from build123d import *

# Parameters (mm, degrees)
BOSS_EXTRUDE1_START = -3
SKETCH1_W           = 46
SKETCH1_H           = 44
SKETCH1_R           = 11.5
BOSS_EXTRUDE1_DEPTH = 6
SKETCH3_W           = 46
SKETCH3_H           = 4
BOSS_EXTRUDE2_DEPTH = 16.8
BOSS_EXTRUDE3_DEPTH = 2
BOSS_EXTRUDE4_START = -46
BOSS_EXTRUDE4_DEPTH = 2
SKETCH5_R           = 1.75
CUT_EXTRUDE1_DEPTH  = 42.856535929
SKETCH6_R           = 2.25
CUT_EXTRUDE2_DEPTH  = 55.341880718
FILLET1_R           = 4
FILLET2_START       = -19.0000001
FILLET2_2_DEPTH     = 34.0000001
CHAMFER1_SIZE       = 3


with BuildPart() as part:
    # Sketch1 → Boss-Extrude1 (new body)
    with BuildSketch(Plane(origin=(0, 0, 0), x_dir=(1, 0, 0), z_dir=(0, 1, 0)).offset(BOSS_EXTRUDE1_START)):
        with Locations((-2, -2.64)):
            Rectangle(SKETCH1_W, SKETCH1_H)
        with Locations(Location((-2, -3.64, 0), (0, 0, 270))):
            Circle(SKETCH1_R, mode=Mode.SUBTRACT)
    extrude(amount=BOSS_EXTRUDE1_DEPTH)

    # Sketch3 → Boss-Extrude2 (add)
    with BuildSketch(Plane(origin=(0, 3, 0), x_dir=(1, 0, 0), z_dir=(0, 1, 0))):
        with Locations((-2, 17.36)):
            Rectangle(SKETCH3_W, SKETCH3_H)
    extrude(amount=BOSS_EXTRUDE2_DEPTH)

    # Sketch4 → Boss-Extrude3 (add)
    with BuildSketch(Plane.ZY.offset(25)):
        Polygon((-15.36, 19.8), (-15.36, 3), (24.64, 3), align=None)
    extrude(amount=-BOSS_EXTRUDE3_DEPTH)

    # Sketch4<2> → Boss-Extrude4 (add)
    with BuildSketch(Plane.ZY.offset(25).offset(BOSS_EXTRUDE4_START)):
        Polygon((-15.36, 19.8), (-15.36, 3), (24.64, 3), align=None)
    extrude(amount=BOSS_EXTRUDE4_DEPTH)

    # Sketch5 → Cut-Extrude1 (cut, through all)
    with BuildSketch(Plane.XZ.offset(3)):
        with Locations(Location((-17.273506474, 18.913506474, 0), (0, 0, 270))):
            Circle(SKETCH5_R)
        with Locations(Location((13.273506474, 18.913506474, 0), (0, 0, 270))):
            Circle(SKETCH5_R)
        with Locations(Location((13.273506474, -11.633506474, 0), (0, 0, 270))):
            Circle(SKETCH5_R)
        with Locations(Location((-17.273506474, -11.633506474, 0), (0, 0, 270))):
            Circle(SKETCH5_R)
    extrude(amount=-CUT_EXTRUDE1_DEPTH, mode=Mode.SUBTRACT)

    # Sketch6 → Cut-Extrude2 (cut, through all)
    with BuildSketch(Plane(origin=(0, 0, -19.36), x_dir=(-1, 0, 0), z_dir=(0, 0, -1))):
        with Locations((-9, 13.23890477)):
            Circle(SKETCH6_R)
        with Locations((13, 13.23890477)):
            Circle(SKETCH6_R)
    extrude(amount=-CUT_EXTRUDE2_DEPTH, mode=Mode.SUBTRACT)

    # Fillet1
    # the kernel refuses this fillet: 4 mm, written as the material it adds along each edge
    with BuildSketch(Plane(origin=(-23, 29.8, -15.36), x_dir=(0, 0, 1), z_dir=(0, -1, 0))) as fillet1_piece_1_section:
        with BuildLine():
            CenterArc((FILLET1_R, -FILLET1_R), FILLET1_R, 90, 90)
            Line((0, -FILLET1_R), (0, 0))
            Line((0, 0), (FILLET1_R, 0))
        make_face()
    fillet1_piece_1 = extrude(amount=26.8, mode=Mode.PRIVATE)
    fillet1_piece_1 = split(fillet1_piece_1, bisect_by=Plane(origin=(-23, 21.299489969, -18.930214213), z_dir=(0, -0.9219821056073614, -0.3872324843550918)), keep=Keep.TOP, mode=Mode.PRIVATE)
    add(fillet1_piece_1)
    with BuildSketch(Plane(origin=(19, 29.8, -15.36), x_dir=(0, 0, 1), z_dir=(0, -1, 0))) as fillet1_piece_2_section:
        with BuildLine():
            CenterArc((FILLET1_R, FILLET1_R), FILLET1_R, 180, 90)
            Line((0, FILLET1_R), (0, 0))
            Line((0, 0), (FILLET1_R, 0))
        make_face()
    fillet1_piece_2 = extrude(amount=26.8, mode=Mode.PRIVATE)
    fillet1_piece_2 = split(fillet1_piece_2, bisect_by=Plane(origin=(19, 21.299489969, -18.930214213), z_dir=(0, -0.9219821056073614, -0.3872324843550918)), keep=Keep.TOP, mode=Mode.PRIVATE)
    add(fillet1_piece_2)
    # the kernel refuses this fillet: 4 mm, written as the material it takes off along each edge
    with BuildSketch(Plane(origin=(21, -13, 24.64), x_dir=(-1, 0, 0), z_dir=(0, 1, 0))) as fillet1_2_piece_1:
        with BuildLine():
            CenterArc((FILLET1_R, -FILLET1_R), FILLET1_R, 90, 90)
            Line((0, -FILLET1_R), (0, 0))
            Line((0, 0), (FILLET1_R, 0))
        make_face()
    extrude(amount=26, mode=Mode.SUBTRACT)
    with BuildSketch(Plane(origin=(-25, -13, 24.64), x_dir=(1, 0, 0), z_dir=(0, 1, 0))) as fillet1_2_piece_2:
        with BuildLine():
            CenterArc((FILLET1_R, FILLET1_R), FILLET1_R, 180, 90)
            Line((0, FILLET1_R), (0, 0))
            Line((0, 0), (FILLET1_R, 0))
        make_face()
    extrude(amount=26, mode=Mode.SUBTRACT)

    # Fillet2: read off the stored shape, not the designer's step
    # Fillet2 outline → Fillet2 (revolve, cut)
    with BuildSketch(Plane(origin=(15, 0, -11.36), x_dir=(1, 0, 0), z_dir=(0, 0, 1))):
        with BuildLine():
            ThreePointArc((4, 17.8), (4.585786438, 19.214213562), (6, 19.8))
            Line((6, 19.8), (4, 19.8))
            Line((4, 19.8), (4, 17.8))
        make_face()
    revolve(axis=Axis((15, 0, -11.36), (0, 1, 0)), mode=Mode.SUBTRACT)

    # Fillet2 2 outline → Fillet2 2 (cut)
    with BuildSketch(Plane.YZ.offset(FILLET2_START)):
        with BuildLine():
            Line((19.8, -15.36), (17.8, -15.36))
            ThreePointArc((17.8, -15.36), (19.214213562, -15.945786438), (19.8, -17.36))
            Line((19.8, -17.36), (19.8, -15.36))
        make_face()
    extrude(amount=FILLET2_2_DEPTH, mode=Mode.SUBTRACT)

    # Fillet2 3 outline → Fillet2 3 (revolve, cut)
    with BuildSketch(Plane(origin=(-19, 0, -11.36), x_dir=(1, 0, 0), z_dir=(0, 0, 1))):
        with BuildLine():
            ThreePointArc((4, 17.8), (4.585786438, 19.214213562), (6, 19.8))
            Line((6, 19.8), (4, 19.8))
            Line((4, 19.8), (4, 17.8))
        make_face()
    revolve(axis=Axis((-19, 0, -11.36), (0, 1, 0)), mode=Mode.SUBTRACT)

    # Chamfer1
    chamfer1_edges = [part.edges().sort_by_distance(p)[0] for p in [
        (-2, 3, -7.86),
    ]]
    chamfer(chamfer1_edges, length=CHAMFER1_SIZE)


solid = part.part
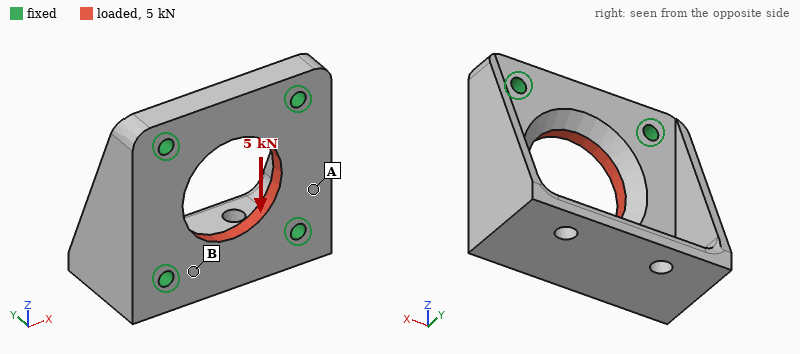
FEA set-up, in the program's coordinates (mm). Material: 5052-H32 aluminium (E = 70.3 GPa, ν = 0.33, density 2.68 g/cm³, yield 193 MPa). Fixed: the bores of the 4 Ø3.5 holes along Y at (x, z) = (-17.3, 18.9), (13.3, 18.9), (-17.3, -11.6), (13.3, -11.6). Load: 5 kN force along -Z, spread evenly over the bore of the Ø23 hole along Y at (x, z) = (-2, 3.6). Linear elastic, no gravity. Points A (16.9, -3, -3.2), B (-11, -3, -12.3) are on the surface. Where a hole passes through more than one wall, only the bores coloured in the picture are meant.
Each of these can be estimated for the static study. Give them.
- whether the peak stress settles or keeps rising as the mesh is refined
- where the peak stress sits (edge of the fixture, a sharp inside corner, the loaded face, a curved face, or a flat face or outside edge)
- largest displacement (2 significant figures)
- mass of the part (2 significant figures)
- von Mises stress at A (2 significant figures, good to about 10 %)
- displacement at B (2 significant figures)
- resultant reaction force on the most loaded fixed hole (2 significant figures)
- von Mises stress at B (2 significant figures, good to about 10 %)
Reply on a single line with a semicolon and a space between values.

keeps rising; edge of the fixture; 11 µm; 36 g; 6.8 MPa; 3.4 µm; 1.3 kN; 21 MPa
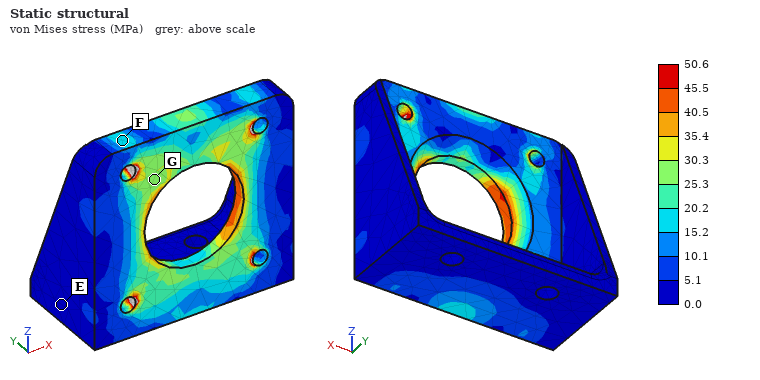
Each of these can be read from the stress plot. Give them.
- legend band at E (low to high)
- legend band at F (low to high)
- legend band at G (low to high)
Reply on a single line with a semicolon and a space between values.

0.0 to 5.1 MPa; 15.2 to 20.2 MPa; 25.3 to 30.3 MPa
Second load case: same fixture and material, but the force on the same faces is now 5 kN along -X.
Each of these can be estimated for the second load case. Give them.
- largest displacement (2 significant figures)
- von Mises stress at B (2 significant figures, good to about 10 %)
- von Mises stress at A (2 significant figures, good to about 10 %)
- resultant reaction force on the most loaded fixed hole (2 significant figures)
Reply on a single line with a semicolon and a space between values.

9.2 µm; 13 MPa; 18 MPa; 1.3 kN
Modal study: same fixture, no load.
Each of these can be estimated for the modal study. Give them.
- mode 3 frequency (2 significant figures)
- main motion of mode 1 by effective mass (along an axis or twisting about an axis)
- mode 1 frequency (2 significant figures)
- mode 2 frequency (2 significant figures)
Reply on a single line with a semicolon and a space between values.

19 kHz; along Z; 11 kHz; 18 kHz
